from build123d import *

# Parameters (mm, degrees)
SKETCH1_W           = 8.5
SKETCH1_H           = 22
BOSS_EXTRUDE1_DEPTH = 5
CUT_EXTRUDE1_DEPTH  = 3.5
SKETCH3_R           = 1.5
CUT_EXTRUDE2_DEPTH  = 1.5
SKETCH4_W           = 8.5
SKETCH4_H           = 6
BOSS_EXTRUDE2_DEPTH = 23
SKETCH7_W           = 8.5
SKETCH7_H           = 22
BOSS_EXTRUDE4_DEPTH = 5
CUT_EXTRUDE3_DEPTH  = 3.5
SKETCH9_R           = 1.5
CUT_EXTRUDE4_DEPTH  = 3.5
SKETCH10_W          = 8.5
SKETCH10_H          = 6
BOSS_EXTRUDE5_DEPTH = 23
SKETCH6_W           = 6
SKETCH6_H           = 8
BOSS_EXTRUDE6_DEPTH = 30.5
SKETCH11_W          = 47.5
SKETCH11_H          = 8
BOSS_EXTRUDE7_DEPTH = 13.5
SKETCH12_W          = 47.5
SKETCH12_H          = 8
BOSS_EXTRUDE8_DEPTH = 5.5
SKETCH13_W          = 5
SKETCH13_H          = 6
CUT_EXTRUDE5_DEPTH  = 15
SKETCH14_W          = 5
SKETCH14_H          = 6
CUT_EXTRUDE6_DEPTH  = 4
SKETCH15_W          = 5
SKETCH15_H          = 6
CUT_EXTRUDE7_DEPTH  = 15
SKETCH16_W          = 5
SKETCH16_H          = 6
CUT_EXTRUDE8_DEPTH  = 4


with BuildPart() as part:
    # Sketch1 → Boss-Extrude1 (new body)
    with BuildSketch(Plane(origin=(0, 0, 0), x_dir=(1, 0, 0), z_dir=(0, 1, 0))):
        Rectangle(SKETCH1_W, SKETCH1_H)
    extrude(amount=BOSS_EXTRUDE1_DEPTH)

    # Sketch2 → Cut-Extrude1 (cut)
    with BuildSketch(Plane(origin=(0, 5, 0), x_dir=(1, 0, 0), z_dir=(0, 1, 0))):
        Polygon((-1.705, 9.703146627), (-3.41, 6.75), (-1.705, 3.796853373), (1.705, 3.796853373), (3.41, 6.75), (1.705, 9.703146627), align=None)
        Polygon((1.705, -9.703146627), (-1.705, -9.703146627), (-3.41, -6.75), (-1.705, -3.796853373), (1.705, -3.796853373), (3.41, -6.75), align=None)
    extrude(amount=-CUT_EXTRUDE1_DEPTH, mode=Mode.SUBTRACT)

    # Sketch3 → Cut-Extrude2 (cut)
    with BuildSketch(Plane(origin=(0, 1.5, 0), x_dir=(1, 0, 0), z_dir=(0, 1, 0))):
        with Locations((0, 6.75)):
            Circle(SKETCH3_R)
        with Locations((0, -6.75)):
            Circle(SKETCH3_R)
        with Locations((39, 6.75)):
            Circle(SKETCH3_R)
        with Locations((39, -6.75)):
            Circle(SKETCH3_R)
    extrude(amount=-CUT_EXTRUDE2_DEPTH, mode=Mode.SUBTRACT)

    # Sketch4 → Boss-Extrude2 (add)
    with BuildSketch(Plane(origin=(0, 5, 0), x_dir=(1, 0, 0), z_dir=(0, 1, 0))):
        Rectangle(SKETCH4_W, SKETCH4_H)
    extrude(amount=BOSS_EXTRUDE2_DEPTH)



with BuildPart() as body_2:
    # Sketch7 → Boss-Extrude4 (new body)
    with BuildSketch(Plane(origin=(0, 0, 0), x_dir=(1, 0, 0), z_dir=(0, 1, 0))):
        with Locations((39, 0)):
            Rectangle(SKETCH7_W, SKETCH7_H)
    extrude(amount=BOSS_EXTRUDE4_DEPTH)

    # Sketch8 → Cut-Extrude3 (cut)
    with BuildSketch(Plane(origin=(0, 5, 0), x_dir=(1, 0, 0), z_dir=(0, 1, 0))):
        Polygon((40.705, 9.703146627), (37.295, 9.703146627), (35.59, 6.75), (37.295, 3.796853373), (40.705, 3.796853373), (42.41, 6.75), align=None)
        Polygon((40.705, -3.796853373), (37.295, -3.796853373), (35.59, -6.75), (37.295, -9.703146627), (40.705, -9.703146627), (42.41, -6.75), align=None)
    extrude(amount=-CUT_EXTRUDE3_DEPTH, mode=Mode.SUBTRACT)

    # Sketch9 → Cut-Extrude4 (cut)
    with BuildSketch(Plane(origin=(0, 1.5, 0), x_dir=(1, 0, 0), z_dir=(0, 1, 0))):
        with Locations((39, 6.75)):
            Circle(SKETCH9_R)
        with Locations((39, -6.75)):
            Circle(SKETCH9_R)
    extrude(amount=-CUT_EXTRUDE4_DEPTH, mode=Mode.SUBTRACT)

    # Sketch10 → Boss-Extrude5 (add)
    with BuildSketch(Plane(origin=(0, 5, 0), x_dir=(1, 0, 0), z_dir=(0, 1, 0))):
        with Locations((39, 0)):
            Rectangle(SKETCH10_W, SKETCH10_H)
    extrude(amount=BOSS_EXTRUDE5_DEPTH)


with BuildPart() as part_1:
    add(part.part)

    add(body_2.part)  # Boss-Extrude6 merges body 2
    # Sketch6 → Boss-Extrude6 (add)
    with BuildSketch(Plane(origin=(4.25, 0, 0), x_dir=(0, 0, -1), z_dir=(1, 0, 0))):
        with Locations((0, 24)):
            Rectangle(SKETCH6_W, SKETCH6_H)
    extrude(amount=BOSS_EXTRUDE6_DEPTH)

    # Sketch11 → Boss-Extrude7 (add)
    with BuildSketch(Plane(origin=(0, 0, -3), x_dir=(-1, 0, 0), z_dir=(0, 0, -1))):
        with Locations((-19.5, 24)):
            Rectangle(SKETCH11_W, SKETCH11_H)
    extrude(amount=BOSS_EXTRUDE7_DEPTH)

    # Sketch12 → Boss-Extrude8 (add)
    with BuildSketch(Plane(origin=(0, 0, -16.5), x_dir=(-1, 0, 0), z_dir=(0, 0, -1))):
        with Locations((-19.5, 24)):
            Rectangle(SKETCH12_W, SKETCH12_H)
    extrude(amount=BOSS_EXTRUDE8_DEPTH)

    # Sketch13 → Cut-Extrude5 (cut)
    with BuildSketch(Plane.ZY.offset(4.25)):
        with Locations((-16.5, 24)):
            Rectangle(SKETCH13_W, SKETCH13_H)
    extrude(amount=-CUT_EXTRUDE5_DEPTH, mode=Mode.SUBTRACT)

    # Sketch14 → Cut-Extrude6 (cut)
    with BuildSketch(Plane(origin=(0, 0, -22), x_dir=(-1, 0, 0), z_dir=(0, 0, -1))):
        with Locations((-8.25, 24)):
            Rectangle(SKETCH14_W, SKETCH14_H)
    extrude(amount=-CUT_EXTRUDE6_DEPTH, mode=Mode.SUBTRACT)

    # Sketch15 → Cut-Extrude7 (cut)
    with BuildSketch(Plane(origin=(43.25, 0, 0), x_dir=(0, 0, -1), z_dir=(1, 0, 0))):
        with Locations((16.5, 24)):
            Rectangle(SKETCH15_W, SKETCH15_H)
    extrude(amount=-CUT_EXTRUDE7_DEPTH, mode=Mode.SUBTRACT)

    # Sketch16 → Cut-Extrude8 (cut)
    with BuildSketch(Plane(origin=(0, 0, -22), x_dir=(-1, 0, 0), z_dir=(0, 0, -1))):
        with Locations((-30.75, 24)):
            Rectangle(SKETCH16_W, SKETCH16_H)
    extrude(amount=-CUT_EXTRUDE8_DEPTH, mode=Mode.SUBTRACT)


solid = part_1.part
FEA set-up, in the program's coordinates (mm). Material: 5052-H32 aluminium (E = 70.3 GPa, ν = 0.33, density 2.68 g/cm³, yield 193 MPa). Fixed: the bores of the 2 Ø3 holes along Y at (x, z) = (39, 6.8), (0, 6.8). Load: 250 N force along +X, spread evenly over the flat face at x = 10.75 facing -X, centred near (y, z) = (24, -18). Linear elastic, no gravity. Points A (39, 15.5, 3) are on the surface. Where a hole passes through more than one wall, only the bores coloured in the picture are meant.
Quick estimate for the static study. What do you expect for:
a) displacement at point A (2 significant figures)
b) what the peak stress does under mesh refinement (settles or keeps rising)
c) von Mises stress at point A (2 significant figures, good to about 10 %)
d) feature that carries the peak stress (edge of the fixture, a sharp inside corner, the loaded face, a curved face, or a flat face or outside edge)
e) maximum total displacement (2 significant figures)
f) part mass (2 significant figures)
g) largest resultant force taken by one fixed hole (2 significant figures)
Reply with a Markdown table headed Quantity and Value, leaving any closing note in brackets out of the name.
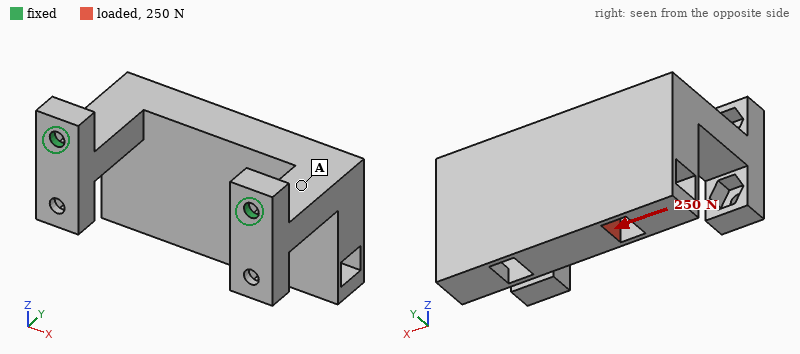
| Quantity | Value |
|---|---|
| displacement at point A | 25 µm |
| what the peak stress does under mesh refinement | keeps rising |
| von Mises stress at point A | 10 MPa |
| feature that carries the peak stress | edge of the fixture |
| maximum total displacement | 59 µm |
| part mass | 30 g |
| largest resultant force taken by one fixed hole | 210 N |
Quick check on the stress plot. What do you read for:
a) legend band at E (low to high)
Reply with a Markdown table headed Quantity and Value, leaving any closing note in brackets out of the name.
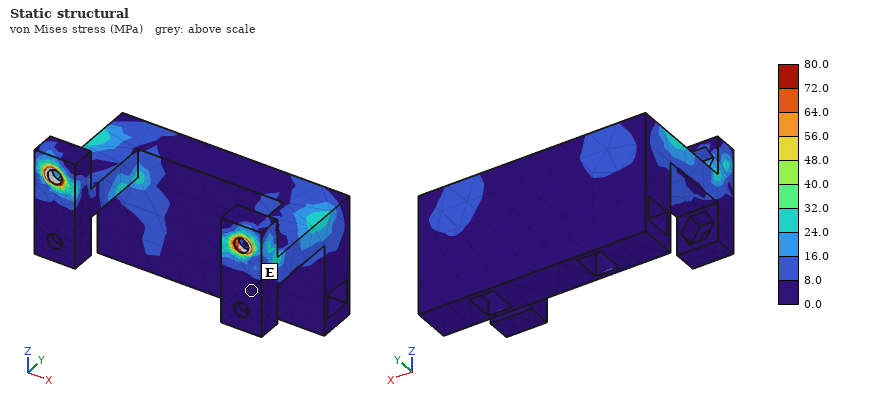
| Quantity | Value |
|---|---|
| legend band at E | 0.0 to 8.0 MPa |
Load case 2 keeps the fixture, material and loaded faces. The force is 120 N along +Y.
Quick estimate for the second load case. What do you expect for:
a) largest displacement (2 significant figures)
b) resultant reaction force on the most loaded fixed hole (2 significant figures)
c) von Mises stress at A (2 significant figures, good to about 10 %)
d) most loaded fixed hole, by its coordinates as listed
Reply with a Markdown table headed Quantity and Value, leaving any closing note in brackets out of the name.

| Quantity | Value |
|---|---|
| largest displacement | 0.25 mm |
| resultant reaction force on the most loaded fixed hole | 87 N |
| von Mises stress at A | 21 MPa |
| most loaded fixed hole, by its coordinates as listed | (0, 6.8) |
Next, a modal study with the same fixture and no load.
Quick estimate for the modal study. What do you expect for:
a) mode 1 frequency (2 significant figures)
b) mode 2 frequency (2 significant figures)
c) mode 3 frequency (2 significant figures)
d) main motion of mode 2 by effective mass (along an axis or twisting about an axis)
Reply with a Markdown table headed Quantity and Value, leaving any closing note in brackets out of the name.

| Quantity | Value |
|---|---|
| mode 1 frequency | 810 Hz |
| mode 2 frequency | 2800 Hz |
| mode 3 frequency | 3300 Hz |
| main motion of mode 2 by effective mass | along X |
